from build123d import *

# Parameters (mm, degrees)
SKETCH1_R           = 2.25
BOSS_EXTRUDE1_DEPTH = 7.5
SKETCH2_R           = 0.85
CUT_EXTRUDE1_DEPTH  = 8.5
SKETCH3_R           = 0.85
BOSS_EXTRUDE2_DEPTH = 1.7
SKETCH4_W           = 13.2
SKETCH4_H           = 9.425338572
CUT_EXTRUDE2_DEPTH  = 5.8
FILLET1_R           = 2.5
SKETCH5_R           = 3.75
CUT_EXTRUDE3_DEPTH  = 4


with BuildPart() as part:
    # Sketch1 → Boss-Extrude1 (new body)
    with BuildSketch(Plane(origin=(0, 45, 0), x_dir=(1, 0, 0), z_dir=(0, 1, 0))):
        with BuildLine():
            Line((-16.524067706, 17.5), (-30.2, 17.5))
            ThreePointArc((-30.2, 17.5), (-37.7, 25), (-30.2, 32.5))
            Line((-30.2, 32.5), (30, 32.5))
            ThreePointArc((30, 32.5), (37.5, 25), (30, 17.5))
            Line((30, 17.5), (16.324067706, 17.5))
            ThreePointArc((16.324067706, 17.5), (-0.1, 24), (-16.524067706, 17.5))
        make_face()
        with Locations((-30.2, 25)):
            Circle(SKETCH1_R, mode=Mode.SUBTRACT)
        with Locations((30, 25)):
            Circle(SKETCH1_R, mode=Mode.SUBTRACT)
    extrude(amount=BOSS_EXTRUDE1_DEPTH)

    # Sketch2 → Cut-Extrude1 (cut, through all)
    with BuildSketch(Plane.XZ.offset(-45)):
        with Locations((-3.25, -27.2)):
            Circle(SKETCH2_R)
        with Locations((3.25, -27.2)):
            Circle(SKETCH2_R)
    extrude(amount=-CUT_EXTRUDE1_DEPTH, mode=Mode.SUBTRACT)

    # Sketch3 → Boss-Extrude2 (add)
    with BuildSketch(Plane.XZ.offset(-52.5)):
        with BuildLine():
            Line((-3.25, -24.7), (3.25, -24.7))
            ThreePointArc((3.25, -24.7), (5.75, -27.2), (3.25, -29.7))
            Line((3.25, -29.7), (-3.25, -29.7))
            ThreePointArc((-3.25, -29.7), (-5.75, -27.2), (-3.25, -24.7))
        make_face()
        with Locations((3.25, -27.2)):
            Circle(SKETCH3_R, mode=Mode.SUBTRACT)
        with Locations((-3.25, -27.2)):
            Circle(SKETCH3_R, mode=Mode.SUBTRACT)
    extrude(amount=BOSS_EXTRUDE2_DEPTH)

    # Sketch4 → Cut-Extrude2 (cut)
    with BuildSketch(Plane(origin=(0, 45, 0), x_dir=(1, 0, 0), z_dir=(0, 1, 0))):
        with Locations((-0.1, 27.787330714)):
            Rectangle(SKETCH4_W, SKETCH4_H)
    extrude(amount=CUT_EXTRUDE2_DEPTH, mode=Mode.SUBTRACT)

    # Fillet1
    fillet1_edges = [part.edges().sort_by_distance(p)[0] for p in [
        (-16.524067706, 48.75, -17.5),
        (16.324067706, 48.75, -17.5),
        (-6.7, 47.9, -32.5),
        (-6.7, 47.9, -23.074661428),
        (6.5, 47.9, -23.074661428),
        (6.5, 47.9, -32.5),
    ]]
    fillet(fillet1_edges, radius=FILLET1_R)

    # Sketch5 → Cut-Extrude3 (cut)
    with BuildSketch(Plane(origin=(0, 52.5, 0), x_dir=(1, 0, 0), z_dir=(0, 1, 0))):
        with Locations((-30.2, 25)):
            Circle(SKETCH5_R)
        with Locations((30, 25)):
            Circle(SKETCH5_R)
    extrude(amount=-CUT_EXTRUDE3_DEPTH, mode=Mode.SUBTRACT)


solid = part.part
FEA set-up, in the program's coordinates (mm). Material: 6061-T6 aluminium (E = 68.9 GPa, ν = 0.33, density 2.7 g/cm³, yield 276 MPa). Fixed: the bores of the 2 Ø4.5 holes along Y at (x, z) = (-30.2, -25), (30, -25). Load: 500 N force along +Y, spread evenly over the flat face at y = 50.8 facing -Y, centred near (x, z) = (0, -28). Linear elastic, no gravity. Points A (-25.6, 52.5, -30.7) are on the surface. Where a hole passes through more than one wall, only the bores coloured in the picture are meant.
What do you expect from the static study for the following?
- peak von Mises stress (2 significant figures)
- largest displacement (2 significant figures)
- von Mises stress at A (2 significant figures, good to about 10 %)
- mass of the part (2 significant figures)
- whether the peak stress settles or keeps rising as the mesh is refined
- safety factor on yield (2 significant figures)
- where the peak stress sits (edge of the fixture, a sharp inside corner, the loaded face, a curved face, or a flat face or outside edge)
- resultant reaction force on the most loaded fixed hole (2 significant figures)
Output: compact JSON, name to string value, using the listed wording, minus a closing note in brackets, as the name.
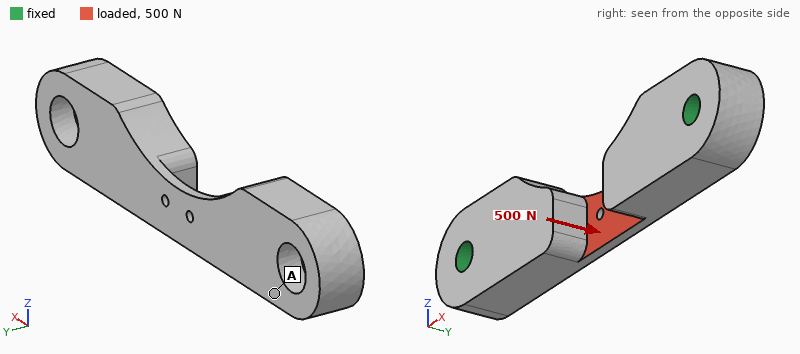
{"peak von Mises stress": "210 MPa", "largest displacement": "76 µm", "von Mises stress at A": "21 MPa", "mass of the part": "16 g", "whether the peak stress settles or keeps rising as the mesh is refined": "settles", "safety factor on yield": "1.3", "where the peak stress sits": "a curved face", "resultant reaction force on the most loaded fixed hole": "630 N"}
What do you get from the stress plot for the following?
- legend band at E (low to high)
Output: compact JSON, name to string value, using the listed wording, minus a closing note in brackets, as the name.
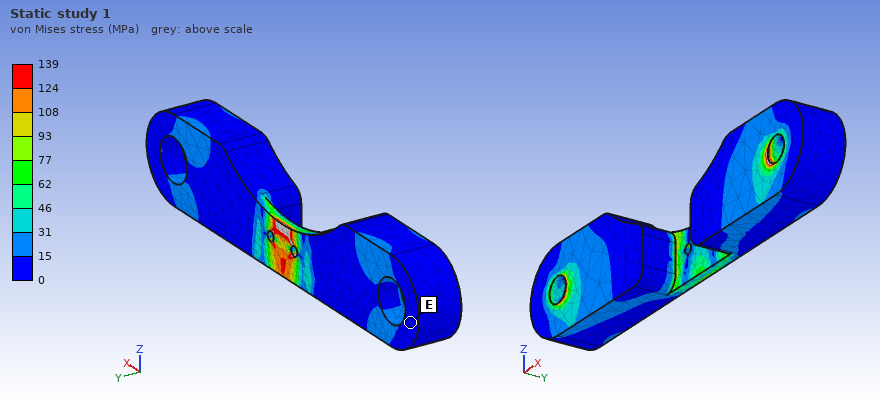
{"legend band at E": "0 to 15 MPa"}
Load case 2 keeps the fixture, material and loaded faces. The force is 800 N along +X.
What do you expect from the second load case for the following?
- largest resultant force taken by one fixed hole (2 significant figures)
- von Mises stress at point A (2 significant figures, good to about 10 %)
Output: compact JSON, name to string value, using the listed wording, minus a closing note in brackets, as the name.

{"largest resultant force taken by one fixed hole": "400 N", "von Mises stress at point A": "13 MPa"}
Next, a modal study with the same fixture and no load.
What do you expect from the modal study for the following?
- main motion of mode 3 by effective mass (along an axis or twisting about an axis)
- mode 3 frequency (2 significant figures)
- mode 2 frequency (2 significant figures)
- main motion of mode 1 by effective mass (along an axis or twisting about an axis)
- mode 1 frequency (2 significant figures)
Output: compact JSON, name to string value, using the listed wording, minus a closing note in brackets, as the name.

{"main motion of mode 3 by effective mass": "along Z", "mode 3 frequency": "11 kHz", "mode 2 frequency": "9500 Hz", "main motion of mode 1 by effective mass": "along Y", "mode 1 frequency": "8600 Hz"}
